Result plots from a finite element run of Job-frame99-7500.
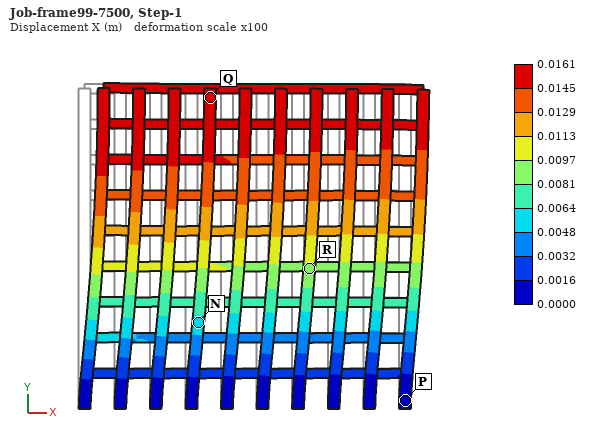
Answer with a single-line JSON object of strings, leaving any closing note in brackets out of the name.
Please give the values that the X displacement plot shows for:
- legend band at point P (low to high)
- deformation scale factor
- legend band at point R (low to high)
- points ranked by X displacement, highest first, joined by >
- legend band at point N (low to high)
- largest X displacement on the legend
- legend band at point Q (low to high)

{"legend band at point P": "0.0000 to 0.0016 m", "deformation scale factor": "100", "legend band at point R": "0.0081 to 0.0097 m", "points ranked by X displacement, highest first, joined by >": "Q > R > N > P", "legend band at point N": "0.0048 to 0.0064 m", "largest X displacement on the legend": "0.0161 m", "legend band at point Q": "0.0145 to 0.0161 m"}
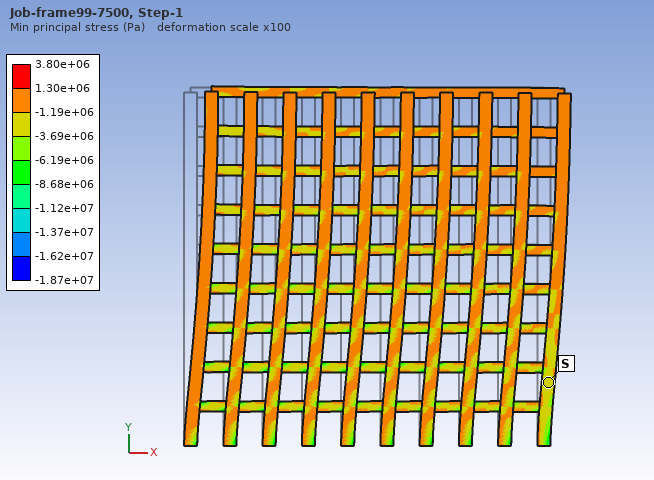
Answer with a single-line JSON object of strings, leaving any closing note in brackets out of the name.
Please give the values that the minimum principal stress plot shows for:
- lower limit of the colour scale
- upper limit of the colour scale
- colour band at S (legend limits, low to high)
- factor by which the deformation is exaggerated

{"lower limit of the colour scale": "-1.87e+07 Pa", "upper limit of the colour scale": "3.80e+06 Pa", "colour band at S": "-3.69e+06 to -1.19e+06 Pa", "factor by which the deformation is exaggerated": "100"}
